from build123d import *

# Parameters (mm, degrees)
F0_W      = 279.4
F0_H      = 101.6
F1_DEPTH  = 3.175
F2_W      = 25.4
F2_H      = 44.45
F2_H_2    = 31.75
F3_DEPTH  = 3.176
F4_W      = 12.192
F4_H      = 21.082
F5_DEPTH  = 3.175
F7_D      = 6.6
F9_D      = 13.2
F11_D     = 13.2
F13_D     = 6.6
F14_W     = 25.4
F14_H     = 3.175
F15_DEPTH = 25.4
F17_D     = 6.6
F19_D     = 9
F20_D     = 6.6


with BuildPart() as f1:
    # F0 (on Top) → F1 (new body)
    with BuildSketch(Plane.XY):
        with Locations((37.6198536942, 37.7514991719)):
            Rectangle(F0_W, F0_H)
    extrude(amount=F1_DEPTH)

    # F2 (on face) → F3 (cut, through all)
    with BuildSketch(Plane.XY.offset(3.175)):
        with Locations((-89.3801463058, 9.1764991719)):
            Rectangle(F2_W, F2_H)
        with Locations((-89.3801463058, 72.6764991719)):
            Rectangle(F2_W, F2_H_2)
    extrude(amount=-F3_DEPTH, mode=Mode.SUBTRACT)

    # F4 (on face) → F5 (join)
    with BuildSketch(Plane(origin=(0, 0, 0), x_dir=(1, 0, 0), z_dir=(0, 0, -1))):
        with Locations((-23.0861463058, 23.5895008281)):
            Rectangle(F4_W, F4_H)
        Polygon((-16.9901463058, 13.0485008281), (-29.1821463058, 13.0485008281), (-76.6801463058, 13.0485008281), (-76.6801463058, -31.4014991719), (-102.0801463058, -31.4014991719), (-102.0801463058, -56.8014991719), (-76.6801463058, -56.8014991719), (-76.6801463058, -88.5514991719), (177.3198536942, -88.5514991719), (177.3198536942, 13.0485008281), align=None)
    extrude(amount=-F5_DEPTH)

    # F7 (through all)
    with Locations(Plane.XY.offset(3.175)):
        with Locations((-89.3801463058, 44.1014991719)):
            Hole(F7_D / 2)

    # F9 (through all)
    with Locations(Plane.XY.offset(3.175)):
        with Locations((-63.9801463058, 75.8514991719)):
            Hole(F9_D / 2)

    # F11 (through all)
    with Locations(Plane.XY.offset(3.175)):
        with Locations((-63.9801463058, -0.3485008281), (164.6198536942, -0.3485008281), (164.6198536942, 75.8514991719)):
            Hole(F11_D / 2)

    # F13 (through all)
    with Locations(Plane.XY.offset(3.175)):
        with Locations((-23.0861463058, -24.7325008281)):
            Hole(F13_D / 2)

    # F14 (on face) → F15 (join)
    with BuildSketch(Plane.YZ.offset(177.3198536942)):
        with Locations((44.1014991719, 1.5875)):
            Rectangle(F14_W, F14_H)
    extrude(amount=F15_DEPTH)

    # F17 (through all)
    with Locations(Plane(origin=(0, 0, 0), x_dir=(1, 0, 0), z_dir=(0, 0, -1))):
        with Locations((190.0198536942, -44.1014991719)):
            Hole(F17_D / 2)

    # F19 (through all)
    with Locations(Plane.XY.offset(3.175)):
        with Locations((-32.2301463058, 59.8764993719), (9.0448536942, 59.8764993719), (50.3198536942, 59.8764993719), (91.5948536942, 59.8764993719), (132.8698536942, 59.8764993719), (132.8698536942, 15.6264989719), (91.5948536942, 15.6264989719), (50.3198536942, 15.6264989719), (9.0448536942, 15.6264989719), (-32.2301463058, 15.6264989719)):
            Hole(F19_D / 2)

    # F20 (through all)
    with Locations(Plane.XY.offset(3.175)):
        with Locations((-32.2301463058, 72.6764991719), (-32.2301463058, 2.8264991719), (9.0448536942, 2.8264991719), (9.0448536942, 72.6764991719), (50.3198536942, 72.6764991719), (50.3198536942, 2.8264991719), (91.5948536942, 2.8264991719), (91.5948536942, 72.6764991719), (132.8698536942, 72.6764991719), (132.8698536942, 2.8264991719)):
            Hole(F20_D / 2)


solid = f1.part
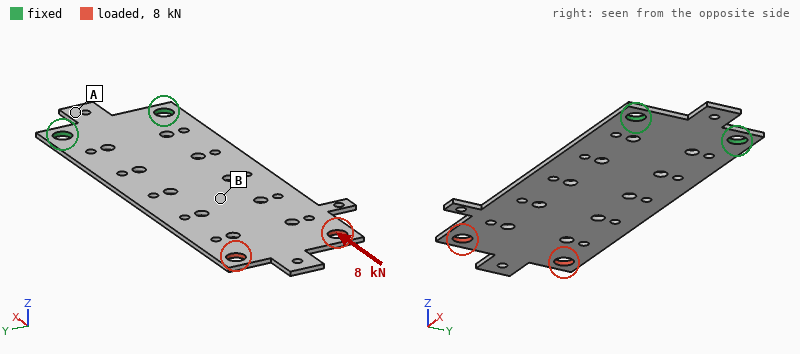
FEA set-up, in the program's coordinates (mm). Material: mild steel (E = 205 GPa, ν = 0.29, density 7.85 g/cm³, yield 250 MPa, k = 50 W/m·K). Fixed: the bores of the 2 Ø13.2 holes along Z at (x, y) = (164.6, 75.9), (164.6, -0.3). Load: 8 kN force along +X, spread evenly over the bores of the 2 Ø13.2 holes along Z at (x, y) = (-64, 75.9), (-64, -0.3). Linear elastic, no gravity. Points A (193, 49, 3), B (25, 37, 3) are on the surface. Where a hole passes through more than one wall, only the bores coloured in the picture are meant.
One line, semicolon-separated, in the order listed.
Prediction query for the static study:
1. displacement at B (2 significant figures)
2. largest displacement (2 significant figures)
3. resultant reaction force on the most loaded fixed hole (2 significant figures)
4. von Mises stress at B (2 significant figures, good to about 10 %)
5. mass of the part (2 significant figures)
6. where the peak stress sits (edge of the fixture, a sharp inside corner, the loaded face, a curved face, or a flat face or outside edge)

21 µm; 42 µm; 4.1 kN; 28 MPa; 640 g; the loaded face
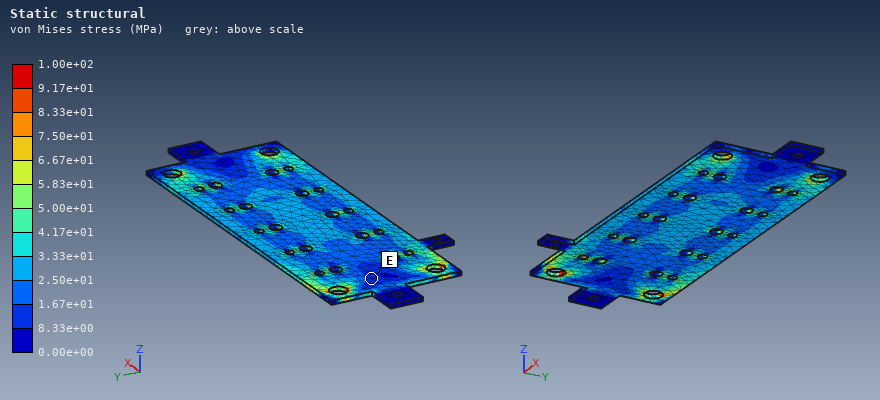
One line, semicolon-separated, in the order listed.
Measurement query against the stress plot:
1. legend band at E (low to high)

8.33e+00 to 1.67e+01 MPa
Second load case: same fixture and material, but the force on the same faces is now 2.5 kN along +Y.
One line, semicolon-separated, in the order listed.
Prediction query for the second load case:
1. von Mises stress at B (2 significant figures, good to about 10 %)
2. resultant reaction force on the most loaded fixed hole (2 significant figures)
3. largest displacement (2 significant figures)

16 MPa; 7.2 kN; 0.27 mm
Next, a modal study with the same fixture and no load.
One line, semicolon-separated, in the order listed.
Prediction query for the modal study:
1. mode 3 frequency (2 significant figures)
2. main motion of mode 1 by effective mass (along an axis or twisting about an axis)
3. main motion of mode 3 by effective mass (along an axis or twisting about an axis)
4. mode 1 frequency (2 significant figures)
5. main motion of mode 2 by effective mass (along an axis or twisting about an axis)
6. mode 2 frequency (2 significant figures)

260 Hz; along Z; along Z; 43 Hz; twisting about X; 220 Hz
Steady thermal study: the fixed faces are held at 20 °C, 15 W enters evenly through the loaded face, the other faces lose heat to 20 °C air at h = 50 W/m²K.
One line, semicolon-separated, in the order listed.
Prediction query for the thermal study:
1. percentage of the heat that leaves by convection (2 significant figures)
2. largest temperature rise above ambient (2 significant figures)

100 %; 42 K
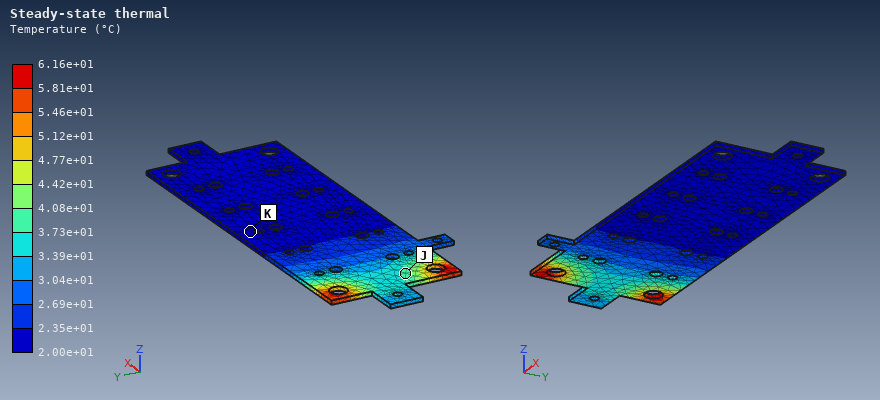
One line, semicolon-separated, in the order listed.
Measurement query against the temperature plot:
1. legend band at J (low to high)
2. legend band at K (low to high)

3.73e+01 to 4.08e+01 °C; 2.00e+01 to 2.35e+01 °C
